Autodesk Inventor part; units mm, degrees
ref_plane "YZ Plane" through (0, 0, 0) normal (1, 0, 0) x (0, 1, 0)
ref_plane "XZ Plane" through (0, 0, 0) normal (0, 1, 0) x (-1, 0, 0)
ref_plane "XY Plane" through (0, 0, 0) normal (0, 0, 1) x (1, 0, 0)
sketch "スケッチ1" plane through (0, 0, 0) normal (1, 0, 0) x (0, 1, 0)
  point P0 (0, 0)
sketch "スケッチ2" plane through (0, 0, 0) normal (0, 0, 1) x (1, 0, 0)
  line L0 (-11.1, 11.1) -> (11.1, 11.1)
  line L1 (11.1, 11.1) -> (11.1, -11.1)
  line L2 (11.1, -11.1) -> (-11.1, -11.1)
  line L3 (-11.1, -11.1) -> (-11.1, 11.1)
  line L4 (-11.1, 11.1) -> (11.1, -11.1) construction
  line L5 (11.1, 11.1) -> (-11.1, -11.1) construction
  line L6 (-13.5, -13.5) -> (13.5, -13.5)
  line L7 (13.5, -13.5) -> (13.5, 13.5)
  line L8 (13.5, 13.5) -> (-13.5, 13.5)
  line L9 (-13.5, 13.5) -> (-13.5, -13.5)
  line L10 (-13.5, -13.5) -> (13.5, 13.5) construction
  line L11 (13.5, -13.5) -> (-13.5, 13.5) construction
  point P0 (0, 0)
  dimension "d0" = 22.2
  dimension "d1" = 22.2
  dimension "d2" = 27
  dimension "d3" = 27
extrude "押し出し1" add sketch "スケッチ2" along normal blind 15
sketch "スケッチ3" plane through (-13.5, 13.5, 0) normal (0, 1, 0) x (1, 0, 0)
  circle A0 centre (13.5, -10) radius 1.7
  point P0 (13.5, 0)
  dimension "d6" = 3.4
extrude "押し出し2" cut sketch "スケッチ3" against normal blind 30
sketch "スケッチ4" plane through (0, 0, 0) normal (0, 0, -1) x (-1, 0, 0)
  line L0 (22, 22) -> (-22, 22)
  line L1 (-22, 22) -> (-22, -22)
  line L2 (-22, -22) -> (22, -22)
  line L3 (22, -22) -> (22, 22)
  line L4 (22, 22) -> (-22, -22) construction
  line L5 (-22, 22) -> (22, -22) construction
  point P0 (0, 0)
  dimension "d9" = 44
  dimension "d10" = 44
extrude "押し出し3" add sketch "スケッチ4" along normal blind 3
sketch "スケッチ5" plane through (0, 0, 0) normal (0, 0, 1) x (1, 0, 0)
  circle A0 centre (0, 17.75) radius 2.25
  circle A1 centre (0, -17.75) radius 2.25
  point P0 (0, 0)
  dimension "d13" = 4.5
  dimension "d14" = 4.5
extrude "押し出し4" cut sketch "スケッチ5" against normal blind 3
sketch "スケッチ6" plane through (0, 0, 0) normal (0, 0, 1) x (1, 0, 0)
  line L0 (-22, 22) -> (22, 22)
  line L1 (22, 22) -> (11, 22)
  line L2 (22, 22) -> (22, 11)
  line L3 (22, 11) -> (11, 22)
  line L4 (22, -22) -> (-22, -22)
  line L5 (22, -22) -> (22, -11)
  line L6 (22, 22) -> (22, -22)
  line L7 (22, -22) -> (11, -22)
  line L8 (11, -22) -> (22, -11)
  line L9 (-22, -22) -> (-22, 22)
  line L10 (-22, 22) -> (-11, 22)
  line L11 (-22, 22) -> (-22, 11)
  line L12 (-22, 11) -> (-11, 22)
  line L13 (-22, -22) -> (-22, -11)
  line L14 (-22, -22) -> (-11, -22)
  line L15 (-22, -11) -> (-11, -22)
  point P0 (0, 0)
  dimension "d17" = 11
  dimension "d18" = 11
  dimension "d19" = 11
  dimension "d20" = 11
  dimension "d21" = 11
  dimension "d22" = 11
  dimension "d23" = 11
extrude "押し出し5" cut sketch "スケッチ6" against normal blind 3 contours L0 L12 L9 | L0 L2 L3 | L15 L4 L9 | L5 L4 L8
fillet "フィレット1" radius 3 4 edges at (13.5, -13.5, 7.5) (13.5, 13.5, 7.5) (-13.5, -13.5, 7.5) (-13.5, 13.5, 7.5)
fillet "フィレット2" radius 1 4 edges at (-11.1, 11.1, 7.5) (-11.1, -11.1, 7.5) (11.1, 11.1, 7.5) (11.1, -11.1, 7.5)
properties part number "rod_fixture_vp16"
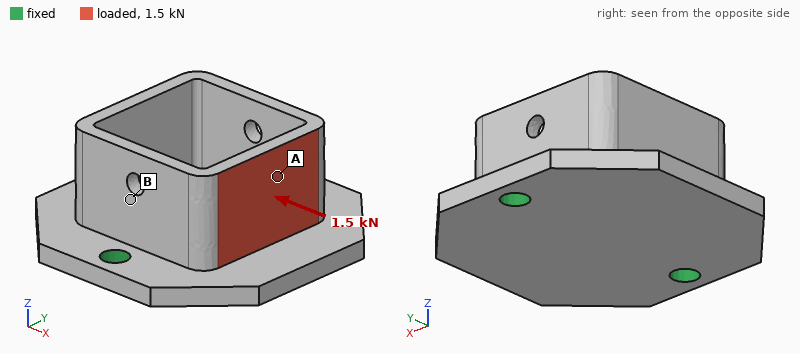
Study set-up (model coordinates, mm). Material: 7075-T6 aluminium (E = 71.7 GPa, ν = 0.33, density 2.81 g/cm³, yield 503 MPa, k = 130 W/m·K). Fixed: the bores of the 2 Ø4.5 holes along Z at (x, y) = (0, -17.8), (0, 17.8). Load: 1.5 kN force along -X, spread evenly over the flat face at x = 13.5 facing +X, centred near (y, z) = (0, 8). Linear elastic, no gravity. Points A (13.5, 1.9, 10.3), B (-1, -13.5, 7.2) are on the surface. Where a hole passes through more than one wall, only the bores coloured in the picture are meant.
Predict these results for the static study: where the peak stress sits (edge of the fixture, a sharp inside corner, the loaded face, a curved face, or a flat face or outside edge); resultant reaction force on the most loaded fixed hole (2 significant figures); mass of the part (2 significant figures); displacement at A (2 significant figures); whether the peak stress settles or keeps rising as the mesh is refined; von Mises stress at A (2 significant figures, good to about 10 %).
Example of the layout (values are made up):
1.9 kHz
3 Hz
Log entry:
edge of the fixture
760 N
24 g
0.14 mm
keeps rising
91 MPa
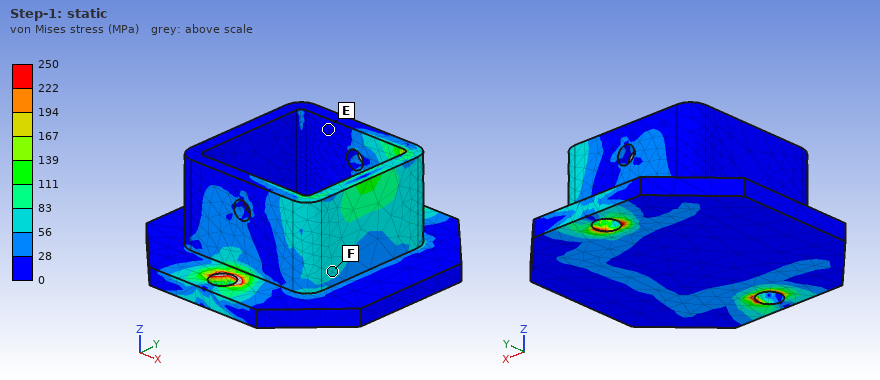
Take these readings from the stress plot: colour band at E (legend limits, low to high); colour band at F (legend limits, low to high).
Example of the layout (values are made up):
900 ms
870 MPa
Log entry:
0 to 28 MPa
56 to 83 MPa
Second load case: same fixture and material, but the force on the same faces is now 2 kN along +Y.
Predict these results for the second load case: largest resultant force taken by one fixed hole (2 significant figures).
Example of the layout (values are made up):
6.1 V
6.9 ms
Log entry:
1.4 kN
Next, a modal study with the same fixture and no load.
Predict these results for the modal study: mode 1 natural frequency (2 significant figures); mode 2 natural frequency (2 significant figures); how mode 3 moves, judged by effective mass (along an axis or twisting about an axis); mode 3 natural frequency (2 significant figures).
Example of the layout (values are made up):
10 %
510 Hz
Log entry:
4300 Hz
9900 Hz
along Z
11 kHz
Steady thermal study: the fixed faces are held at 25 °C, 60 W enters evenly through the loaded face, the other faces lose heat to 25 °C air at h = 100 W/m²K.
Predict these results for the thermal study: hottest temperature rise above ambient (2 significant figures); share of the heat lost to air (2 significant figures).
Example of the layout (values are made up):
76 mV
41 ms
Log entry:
77 K
24 %
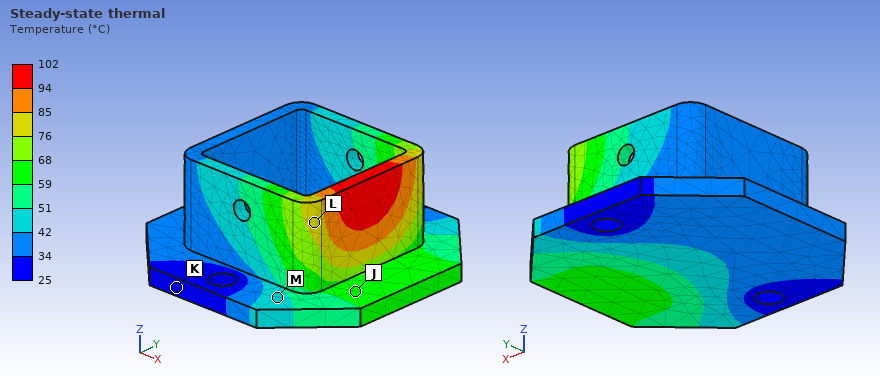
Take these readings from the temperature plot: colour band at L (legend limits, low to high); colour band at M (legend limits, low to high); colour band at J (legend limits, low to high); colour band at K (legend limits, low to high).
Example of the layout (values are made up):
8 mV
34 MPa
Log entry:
76 to 85 °C
42 to 51 °C
59 to 68 °C
25 to 34 °C
